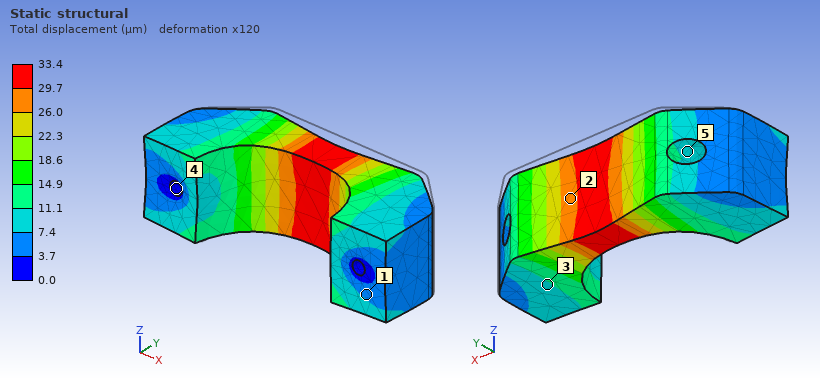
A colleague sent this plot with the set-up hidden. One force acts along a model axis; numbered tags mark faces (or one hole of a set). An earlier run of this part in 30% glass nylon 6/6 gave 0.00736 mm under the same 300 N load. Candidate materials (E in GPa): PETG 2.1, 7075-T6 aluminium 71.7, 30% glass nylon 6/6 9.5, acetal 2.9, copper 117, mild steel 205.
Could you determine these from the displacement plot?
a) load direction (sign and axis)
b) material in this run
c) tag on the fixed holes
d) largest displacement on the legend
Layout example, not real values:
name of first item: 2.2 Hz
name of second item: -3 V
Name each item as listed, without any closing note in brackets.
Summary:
load direction: -Y
material in this run: PETG
tag on the fixed holes: 4
largest displacement on the legend: 33.4 µm
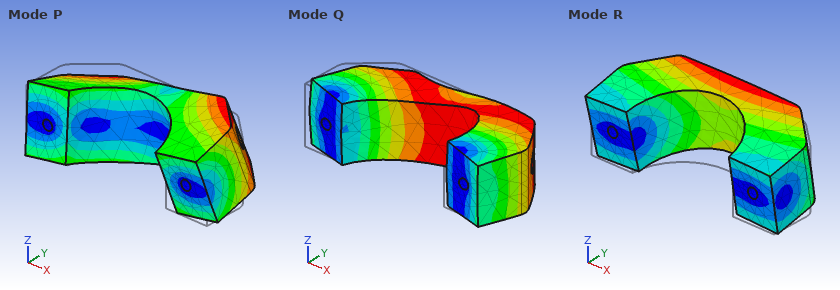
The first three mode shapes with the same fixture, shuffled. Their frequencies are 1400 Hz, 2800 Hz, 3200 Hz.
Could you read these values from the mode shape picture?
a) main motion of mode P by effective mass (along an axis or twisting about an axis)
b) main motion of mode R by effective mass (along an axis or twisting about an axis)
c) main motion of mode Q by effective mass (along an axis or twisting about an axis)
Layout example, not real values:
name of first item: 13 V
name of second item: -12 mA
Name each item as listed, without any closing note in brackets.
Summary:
main motion of mode P by effective mass: twisting about Y
main motion of mode R by effective mass: along Z
main motion of mode Q by effective mass: along X
